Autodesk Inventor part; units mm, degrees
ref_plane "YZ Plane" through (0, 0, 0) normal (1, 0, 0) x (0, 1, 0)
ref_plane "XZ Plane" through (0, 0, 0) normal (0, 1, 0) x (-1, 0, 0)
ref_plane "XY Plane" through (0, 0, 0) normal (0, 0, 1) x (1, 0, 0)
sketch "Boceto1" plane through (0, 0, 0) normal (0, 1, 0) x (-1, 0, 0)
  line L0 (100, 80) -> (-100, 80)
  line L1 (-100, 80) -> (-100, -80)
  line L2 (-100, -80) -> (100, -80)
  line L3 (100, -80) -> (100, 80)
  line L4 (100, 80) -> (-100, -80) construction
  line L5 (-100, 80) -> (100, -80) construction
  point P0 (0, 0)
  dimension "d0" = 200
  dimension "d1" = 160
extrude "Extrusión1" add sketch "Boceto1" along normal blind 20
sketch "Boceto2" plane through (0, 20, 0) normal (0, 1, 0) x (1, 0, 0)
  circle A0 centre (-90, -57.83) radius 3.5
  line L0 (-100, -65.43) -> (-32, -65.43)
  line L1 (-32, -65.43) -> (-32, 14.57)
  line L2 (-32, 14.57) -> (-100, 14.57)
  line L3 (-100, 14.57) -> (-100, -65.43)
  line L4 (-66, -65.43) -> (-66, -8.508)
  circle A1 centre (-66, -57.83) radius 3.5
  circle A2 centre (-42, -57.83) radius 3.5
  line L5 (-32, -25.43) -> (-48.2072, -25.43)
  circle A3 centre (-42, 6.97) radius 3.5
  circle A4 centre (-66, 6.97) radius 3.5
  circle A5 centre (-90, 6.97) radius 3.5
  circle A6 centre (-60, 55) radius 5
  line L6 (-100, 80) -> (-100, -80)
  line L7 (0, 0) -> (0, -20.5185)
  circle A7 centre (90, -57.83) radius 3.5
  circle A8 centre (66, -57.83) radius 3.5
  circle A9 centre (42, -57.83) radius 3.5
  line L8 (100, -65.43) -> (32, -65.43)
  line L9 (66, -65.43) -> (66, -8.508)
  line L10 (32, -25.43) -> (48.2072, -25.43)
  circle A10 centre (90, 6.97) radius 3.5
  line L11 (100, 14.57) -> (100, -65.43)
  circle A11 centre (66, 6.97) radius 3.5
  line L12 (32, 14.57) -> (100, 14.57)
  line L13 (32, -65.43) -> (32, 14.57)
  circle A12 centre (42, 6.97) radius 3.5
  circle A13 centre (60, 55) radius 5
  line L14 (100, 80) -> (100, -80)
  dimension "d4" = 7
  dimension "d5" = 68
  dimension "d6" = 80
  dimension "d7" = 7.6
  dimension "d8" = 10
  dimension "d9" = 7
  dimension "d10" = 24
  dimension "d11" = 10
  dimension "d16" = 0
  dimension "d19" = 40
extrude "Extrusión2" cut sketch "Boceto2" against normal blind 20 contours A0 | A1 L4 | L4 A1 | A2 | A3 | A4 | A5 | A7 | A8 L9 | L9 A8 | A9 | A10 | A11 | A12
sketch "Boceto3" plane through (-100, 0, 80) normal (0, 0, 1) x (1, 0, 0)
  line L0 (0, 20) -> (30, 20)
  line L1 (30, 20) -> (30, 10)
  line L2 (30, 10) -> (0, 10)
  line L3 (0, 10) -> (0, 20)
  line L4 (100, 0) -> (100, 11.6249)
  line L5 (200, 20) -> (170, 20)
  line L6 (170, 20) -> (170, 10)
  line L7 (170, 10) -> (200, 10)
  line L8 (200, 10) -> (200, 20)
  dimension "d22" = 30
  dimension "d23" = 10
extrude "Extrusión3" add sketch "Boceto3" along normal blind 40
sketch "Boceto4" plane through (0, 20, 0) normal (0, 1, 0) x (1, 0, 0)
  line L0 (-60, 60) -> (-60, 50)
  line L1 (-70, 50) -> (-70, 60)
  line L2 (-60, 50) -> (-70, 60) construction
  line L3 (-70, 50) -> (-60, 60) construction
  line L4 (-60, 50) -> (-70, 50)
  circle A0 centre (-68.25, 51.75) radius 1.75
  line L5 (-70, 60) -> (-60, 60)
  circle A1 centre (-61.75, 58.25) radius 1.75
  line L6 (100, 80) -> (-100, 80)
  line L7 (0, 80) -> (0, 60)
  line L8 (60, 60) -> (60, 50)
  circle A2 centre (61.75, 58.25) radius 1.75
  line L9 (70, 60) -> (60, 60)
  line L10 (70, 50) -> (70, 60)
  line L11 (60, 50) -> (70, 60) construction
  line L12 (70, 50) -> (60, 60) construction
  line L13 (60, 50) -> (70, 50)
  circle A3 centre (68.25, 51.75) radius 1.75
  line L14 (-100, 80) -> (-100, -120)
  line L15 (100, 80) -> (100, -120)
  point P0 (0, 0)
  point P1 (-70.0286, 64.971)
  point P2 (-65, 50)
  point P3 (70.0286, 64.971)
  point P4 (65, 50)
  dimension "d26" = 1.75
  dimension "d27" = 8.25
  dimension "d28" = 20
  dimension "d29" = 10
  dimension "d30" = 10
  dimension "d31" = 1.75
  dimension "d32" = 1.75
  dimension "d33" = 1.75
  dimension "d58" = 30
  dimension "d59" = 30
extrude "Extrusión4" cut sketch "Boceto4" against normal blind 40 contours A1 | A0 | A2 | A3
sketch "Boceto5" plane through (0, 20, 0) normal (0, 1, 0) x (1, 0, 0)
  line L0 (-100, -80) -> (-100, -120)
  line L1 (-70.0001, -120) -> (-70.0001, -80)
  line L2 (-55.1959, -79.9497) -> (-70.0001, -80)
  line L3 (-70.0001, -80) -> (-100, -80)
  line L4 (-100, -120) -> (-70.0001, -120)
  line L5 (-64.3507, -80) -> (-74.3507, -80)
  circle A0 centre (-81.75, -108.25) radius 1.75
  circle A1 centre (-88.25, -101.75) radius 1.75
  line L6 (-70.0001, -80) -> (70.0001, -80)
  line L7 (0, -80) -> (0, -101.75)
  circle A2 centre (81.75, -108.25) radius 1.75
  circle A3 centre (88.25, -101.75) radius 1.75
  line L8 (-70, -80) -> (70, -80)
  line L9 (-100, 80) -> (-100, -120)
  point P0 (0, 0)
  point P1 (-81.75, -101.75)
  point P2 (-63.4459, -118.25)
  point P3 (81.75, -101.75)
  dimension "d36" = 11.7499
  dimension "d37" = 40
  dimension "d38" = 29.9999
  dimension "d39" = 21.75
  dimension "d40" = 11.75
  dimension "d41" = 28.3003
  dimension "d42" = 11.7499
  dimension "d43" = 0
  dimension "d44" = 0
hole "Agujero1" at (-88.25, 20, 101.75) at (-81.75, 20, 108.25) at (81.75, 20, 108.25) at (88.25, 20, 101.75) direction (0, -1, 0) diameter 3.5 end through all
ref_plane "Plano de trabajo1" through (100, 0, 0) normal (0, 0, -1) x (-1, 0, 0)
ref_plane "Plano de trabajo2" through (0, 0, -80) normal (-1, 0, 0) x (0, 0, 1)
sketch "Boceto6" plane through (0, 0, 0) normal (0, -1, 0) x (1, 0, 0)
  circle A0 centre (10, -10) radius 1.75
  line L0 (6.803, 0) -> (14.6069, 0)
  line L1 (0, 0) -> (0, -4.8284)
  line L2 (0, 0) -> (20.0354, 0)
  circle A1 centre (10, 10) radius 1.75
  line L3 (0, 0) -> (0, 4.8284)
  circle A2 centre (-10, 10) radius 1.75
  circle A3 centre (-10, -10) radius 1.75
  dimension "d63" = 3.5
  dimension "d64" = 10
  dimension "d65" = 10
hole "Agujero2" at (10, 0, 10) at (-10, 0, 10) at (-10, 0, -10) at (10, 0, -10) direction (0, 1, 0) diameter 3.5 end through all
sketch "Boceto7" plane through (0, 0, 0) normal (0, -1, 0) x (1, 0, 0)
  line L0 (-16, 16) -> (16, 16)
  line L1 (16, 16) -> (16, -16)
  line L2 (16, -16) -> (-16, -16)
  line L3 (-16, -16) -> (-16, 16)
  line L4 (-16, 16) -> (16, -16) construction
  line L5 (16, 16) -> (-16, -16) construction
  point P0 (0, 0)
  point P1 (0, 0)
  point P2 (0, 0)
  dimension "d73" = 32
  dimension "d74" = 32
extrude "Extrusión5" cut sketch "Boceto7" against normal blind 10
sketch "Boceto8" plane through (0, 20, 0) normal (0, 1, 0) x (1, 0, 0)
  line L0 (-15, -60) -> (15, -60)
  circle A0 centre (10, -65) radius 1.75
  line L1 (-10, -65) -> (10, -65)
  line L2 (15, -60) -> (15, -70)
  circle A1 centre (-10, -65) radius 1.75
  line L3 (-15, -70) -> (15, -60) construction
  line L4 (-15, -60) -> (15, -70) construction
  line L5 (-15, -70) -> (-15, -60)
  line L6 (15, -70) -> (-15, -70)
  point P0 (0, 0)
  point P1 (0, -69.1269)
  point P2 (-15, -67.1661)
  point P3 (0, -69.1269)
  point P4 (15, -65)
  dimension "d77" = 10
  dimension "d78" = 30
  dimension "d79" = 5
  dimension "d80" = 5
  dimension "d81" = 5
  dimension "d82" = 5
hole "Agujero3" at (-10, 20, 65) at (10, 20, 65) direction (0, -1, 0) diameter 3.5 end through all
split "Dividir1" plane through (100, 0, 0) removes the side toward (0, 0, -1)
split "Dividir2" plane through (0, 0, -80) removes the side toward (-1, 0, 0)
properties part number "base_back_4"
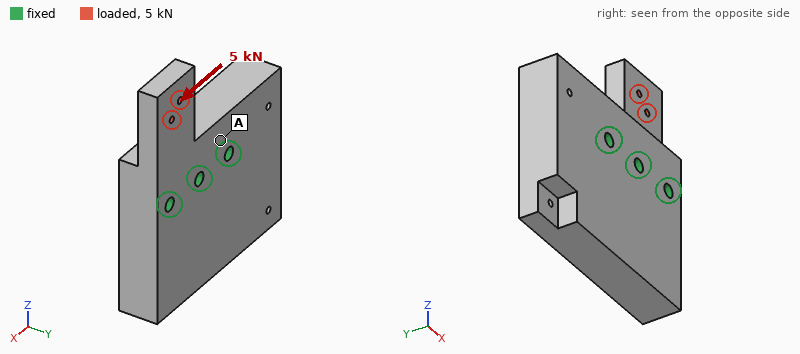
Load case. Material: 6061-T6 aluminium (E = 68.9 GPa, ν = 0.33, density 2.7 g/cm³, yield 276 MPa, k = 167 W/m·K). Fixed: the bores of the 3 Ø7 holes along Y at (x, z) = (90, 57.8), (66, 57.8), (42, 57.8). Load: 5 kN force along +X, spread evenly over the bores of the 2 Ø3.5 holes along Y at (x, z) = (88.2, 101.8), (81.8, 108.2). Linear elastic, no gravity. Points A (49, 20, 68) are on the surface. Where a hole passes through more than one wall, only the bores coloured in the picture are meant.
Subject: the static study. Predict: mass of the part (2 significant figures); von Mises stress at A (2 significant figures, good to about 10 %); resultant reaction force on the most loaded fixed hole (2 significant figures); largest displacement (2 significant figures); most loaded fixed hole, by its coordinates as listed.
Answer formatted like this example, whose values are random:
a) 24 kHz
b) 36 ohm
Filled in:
a) 450 g
b) 10 MPa
c) 6.7 kN
d) 0.11 mm
e) (90, 57.8)
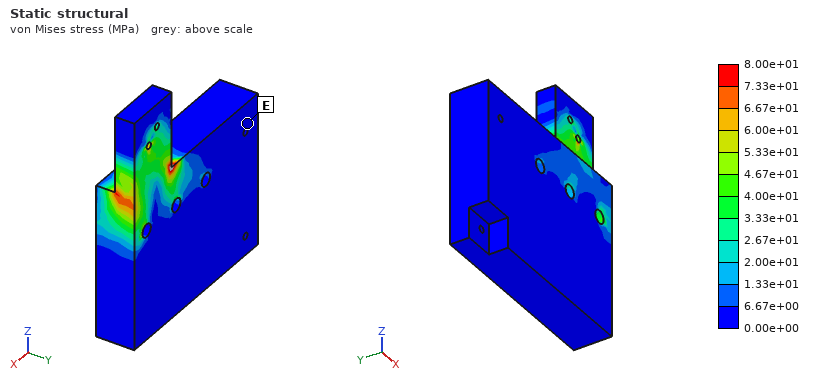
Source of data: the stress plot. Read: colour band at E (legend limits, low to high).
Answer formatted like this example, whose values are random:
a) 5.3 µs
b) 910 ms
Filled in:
a) 0.00e+00 to 6.67e+00 MPa
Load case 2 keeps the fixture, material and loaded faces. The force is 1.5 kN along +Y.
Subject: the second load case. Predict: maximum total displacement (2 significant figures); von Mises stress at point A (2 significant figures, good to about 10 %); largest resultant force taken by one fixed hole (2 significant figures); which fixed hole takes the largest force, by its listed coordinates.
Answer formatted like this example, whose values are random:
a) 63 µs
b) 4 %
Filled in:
a) 0.16 mm
b) 5.0 MPa
c) 900 N
d) (90, 57.8)
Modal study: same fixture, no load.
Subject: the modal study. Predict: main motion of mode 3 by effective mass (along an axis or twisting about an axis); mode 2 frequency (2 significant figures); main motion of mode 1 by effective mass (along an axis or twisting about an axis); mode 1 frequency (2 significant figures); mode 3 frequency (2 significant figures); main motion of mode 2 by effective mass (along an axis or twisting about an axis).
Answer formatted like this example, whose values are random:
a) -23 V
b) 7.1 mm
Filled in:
a) twisting about Z
b) 4000 Hz
c) twisting about X
d) 3700 Hz
e) 5600 Hz
f) along Y
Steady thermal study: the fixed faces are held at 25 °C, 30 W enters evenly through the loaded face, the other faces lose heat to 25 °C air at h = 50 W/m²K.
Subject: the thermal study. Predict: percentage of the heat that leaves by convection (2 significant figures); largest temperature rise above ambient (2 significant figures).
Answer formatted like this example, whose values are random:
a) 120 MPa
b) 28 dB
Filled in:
a) 10 %
b) 22 K
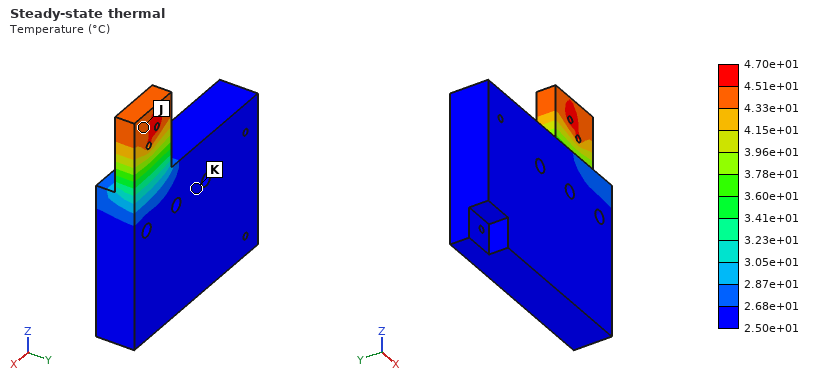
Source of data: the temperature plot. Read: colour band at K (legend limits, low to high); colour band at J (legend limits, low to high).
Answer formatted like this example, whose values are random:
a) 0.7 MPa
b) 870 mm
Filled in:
a) 2.50e+01 to 2.68e+01 °C
b) 4.33e+01 to 4.51e+01 °C
